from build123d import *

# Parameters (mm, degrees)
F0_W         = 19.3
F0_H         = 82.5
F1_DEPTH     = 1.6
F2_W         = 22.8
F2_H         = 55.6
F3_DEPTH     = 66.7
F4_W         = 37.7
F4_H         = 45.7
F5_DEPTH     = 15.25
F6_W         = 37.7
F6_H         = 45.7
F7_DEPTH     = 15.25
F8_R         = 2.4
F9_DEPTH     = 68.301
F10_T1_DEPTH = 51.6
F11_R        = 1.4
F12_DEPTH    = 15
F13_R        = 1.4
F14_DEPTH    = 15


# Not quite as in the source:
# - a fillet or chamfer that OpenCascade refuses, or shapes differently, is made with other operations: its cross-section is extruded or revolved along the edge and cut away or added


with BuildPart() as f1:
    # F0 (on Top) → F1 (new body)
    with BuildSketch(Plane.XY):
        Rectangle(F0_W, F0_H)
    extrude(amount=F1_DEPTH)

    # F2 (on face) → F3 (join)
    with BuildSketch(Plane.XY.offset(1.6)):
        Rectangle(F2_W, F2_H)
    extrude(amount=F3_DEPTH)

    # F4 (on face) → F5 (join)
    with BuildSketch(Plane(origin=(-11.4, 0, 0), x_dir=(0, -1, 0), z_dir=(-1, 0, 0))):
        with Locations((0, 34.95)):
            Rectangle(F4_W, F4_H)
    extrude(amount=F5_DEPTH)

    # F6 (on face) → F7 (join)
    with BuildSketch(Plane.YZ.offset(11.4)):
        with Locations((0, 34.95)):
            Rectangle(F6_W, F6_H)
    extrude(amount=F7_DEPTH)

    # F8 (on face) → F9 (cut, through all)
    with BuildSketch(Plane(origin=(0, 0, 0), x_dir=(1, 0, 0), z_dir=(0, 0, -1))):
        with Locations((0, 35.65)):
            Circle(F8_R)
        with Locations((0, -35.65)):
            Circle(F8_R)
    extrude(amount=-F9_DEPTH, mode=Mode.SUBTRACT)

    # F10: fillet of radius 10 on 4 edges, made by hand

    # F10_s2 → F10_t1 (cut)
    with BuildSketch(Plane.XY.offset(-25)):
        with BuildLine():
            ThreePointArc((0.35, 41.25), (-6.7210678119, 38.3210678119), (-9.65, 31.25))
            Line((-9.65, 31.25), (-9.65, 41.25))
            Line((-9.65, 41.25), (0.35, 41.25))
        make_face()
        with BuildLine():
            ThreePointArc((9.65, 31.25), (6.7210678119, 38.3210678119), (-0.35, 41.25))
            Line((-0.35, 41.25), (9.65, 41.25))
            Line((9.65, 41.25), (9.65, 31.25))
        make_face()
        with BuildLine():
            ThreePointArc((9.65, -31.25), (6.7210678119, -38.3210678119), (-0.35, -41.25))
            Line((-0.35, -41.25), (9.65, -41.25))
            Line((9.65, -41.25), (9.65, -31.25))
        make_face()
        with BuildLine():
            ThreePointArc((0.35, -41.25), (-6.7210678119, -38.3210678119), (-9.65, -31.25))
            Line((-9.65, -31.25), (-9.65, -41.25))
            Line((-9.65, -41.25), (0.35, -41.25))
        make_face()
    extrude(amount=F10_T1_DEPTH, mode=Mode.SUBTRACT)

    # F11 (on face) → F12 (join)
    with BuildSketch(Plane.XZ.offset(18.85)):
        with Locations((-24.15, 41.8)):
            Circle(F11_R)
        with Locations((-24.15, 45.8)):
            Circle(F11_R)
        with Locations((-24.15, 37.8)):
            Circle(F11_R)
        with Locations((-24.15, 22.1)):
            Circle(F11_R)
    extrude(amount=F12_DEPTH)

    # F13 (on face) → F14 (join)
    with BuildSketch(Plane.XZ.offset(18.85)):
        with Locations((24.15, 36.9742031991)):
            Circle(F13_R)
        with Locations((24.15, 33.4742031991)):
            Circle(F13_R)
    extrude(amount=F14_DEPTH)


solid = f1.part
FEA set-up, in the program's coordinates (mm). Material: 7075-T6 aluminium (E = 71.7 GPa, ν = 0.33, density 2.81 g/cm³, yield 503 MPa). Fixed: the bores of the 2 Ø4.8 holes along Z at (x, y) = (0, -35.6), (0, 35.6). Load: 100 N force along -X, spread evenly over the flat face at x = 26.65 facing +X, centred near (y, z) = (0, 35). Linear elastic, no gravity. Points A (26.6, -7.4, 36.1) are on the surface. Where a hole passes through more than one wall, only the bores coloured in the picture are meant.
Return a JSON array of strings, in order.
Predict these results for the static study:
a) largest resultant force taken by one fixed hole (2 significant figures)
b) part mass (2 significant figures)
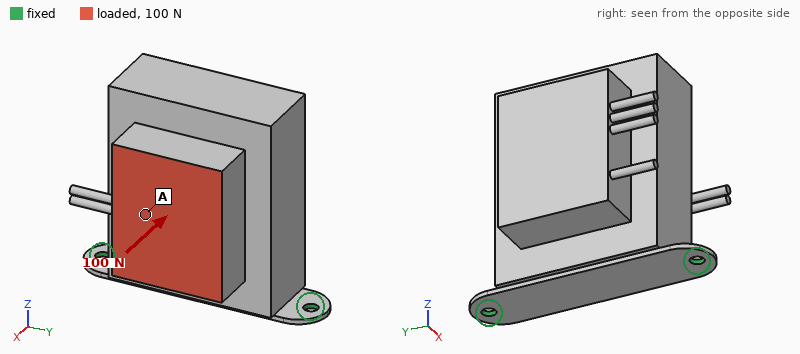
["50 N", "390 g"]
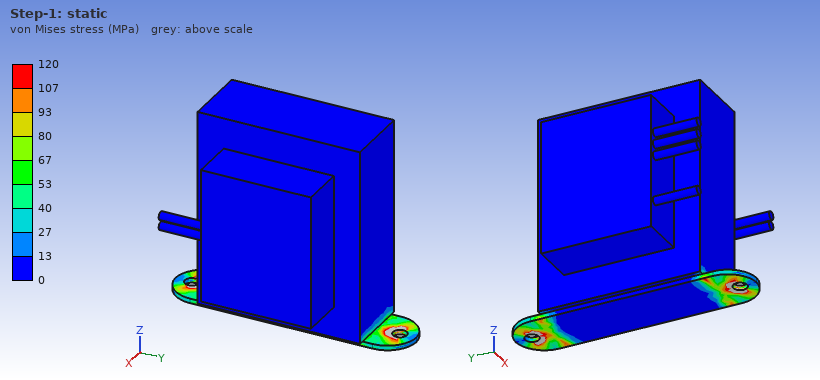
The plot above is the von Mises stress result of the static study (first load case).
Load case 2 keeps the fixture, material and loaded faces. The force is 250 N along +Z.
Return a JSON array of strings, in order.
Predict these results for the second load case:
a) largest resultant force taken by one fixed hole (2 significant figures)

["140 N"]
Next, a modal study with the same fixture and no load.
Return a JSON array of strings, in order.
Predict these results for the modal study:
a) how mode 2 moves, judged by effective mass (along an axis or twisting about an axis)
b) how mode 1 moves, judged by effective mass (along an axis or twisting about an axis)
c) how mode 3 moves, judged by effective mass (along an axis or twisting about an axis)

["along Y", "along X", "along Z"]
